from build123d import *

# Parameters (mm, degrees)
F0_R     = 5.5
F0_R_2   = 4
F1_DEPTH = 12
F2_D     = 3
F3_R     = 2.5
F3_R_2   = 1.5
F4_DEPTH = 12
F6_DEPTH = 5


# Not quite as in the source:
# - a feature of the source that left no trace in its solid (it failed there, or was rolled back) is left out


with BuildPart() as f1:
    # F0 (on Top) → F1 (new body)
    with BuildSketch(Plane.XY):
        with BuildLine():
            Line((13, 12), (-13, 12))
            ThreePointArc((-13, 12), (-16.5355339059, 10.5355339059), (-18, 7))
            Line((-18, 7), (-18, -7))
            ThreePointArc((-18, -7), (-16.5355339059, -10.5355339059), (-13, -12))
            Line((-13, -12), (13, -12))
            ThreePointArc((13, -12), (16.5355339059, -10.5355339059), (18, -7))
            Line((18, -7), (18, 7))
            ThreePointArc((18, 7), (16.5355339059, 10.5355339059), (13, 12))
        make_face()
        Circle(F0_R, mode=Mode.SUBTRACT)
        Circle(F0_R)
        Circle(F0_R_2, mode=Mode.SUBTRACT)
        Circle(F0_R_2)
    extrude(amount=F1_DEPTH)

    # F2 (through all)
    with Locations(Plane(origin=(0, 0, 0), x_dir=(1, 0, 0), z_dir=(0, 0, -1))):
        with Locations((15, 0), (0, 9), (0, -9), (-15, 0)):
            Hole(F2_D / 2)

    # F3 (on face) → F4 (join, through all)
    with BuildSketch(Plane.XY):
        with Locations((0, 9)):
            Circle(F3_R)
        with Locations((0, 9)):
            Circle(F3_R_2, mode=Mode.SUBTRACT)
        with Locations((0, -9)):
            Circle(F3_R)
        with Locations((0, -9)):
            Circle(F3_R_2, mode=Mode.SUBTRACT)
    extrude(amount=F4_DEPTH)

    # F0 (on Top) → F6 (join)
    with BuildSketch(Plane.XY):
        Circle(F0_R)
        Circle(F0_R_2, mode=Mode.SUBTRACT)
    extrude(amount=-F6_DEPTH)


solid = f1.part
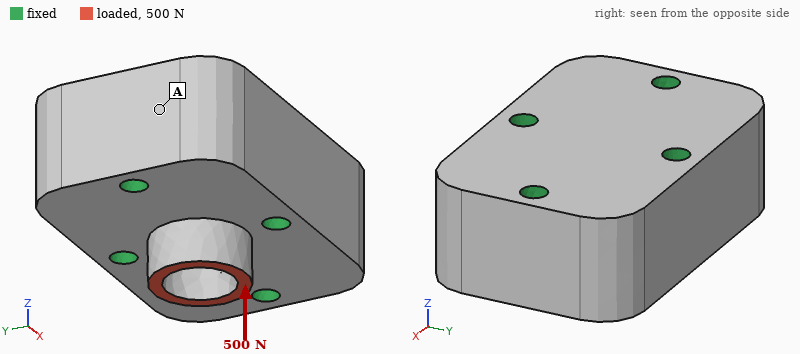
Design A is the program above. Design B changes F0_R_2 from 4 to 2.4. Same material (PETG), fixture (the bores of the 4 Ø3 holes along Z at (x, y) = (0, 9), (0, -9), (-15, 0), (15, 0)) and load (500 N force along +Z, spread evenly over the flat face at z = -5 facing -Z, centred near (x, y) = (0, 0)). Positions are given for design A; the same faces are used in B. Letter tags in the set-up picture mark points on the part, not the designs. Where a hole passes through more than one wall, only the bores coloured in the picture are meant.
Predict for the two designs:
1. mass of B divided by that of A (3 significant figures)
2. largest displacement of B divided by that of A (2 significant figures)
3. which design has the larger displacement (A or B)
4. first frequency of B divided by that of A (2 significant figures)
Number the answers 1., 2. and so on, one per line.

1. 1.02
2. 0.68
3. A
4. 1.00
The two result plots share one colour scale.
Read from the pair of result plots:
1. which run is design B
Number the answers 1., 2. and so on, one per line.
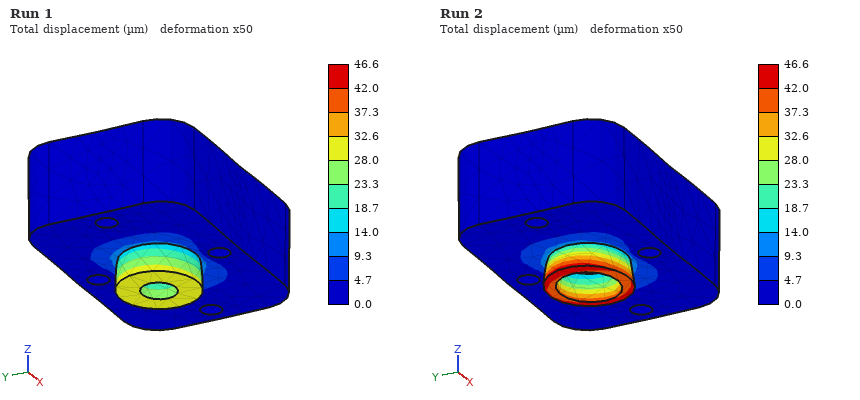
1. Run 1
